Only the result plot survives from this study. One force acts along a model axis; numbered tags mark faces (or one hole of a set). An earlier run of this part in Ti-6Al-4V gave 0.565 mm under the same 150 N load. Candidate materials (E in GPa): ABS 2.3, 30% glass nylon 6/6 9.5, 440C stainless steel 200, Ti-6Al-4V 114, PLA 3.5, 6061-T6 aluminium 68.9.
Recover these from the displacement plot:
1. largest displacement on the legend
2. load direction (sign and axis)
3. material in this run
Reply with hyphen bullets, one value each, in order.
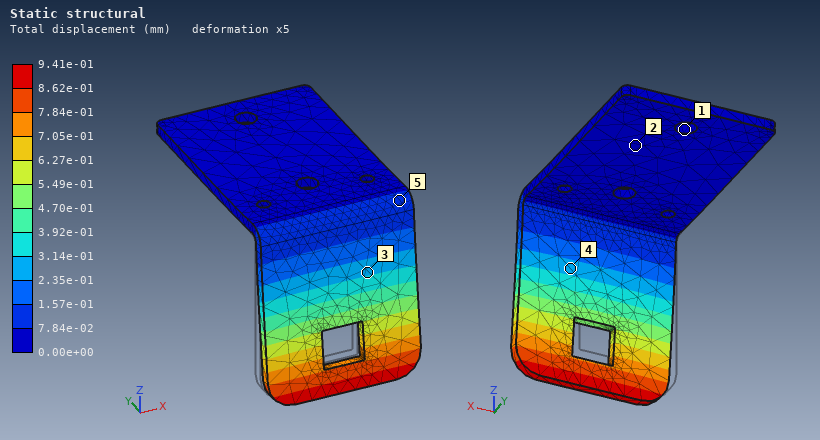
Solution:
- 9.41e-01 mm
- -Y
- 6061-T6 aluminium
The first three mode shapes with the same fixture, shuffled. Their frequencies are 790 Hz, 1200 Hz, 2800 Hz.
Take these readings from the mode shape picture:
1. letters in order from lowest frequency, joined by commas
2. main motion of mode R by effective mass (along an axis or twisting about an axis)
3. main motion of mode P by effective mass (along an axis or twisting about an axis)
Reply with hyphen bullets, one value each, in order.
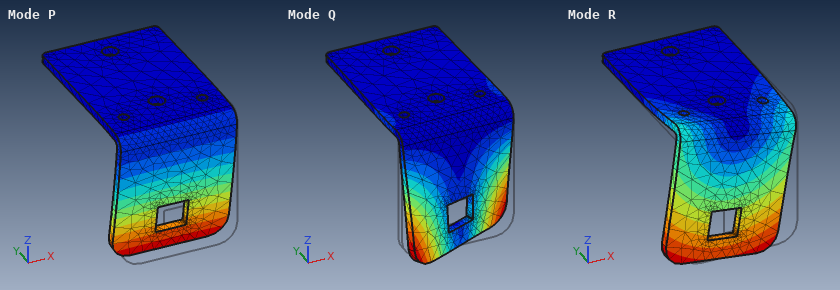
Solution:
- P, R, Q
- along X
- along Y
